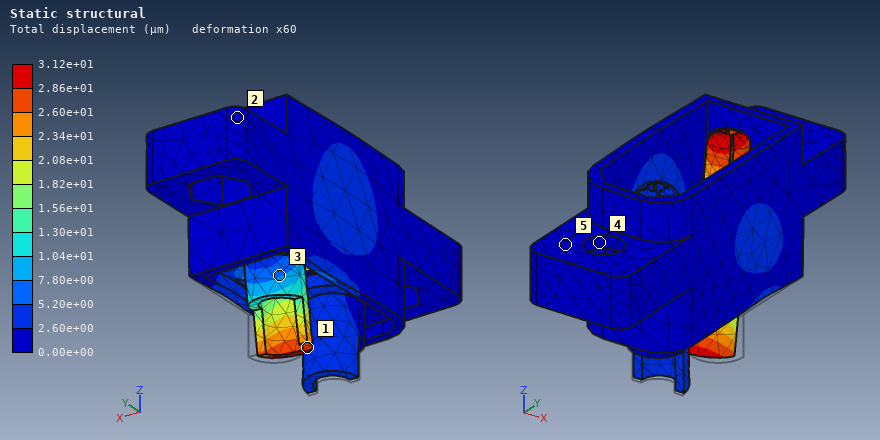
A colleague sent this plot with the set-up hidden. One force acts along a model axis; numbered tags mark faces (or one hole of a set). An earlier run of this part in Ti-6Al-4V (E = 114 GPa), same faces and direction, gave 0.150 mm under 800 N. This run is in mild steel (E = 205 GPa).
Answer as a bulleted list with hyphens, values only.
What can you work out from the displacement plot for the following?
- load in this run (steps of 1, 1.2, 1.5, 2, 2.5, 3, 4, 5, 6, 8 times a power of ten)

- 300 N
